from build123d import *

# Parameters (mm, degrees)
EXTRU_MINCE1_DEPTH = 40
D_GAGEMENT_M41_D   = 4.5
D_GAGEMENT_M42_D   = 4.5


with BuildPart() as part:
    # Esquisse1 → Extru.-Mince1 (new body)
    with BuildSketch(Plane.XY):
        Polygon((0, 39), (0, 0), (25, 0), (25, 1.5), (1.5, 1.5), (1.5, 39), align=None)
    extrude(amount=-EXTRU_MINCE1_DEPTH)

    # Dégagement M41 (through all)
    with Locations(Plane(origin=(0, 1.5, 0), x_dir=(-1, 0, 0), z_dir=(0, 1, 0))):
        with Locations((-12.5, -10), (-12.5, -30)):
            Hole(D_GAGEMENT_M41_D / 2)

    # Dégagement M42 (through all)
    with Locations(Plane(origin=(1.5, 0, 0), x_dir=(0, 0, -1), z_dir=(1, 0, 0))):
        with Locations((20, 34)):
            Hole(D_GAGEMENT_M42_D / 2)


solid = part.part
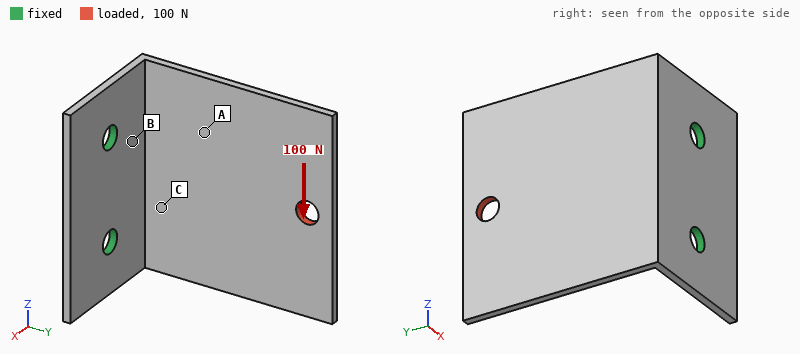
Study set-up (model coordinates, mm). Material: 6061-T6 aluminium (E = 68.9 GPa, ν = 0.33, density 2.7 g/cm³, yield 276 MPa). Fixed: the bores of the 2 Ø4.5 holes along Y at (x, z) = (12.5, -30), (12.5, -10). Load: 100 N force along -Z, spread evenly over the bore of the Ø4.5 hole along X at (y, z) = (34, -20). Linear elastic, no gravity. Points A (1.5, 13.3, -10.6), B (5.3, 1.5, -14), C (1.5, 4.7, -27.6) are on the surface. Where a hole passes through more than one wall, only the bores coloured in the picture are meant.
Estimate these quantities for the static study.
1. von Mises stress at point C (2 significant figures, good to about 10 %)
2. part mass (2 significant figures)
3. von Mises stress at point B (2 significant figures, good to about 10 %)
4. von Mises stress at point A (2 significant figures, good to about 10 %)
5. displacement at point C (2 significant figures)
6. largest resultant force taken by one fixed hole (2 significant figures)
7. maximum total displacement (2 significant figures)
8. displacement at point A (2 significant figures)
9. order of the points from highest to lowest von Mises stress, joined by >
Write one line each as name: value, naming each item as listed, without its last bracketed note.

von Mises stress at point C: 45 MPa
part mass: 9.9 g
von Mises stress at point B: 69 MPa
von Mises stress at point A: 21 MPa
displacement at point C: 0.065 mm
largest resultant force taken by one fixed hole: 150 N
maximum total displacement: 0.36 mm
displacement at point A: 0.13 mm
order of the points from highest to lowest von Mises stress, joined by >: B > C > A
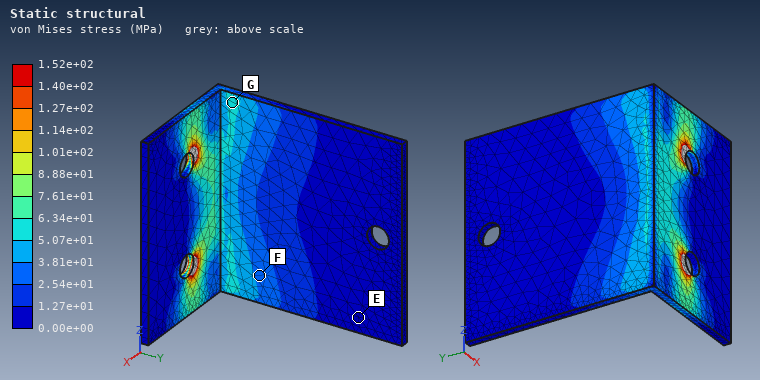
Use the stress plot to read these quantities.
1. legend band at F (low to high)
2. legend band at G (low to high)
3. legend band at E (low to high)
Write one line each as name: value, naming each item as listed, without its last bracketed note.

legend band at F: 2.54e+01 to 3.81e+01 MPa
legend band at G: 5.07e+01 to 6.34e+01 MPa
legend band at E: 0.00e+00 to 1.27e+01 MPa
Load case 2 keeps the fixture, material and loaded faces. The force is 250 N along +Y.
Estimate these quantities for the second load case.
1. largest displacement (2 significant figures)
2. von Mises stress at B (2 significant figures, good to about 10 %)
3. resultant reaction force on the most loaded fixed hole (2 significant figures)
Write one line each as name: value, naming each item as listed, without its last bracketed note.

largest displacement: 0.70 mm
von Mises stress at B: 73 MPa
resultant reaction force on the most loaded fixed hole: 130 N
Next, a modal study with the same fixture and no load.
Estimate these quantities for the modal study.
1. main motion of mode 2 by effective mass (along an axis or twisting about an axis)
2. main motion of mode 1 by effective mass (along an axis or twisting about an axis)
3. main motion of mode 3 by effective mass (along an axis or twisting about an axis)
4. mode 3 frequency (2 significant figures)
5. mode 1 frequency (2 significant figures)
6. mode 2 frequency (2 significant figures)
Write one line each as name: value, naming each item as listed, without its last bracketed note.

main motion of mode 2 by effective mass: along Z
main motion of mode 1 by effective mass: along X
main motion of mode 3 by effective mass: along Z
mode 3 frequency: 2100 Hz
mode 1 frequency: 600 Hz
mode 2 frequency: 1500 Hz
